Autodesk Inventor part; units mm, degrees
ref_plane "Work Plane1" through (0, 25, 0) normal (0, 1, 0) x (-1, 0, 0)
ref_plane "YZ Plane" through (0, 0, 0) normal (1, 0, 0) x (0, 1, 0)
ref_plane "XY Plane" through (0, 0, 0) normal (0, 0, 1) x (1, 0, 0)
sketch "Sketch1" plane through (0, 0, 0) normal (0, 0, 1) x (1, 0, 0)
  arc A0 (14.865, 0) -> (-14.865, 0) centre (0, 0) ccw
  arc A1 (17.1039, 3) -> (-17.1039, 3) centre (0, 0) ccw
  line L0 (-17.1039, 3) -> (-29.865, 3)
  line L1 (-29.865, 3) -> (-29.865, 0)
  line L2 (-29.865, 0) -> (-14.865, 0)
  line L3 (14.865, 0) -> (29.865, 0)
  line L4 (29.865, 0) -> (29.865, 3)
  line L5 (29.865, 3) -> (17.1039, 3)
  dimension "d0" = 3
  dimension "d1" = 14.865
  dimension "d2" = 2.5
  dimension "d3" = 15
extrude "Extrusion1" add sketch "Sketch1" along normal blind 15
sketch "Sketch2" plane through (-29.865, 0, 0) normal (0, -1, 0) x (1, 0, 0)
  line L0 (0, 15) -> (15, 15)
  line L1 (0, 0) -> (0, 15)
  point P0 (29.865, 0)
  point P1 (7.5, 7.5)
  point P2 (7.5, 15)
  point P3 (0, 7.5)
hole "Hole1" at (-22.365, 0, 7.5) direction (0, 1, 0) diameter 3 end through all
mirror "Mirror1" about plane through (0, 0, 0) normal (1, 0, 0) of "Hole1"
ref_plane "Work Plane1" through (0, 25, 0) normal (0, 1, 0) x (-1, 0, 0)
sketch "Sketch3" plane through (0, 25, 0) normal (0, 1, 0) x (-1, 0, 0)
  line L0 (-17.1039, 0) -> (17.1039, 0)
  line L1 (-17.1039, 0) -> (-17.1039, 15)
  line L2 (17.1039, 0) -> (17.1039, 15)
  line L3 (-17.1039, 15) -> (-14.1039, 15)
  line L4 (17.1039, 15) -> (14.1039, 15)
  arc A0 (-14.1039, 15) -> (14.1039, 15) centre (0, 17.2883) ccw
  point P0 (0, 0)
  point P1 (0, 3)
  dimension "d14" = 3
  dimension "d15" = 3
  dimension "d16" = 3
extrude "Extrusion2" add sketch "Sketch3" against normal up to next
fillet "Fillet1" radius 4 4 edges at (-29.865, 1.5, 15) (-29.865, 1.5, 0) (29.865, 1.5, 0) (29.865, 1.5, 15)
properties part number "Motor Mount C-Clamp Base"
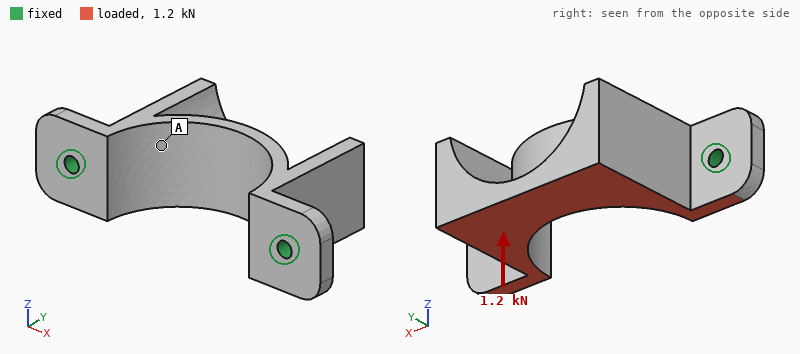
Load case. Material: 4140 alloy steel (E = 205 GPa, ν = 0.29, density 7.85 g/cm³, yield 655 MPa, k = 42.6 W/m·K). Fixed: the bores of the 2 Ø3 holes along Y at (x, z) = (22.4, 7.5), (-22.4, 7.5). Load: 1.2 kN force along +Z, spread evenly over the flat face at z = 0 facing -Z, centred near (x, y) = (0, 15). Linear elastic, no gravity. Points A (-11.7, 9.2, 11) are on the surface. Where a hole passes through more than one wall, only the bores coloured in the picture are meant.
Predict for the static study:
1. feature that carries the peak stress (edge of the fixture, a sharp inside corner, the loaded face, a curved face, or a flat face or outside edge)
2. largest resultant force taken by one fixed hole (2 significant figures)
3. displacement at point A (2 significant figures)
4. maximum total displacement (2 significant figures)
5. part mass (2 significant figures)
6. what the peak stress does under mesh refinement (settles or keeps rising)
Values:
edge of the fixture
600 N
0.044 mm
0.12 mm
50 g
keeps rising
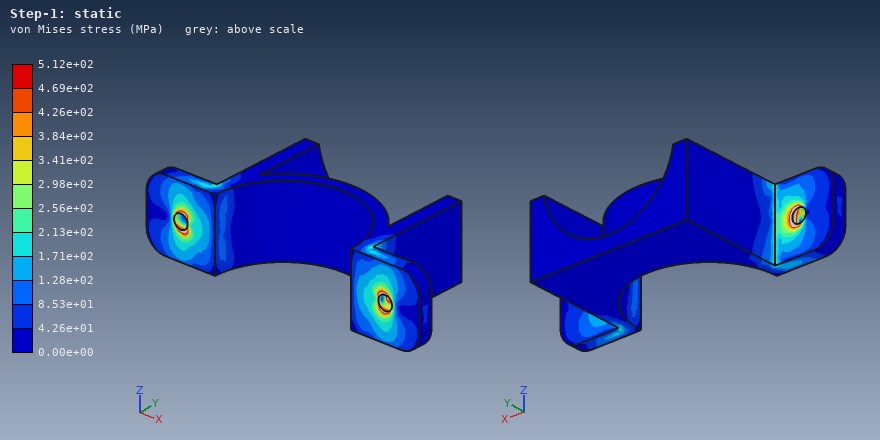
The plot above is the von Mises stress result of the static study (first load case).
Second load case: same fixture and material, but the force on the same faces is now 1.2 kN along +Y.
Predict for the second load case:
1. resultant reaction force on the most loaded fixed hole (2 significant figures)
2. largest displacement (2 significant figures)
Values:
660 N
62 µm
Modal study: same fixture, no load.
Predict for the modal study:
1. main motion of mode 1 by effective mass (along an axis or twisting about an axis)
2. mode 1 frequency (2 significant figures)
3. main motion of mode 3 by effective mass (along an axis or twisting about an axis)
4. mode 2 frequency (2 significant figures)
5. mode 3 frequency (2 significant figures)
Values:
along Z
2900 Hz
along X
6400 Hz
10000 Hz
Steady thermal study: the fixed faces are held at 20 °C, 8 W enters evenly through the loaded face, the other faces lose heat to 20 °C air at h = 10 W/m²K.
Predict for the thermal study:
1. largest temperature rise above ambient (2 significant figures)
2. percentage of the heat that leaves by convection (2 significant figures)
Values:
33 K
8.8 %
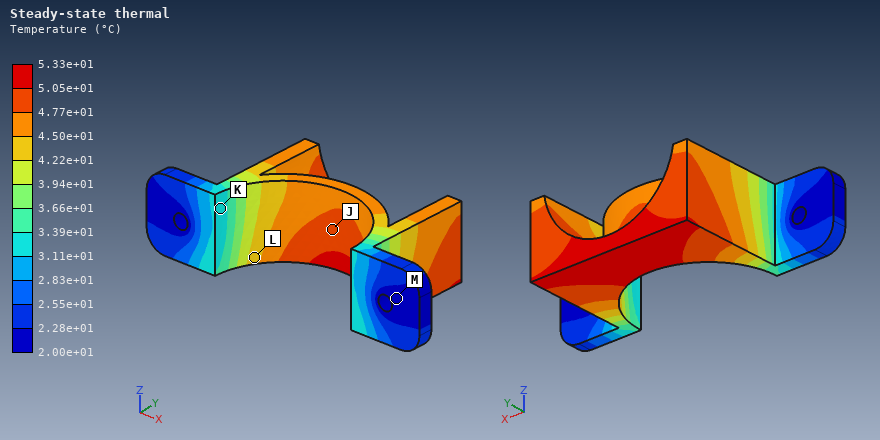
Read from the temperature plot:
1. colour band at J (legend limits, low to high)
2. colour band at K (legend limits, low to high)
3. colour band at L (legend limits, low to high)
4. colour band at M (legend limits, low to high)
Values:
4.77e+01 to 5.05e+01 °C
3.11e+01 to 3.39e+01 °C
4.22e+01 to 4.50e+01 °C
2.00e+01 to 2.28e+01 °C
